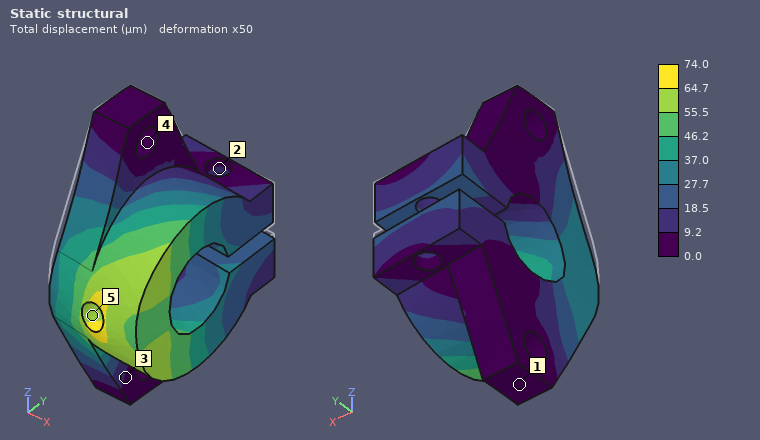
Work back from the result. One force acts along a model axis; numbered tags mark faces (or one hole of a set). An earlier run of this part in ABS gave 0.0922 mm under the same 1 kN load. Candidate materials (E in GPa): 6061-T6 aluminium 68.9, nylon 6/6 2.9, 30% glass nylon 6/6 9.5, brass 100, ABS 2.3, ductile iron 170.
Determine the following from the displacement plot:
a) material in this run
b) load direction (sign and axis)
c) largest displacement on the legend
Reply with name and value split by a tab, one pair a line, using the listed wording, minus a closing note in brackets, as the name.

material in this run	nylon 6/6
load direction	-Z
largest displacement on the legend	74.0 µm
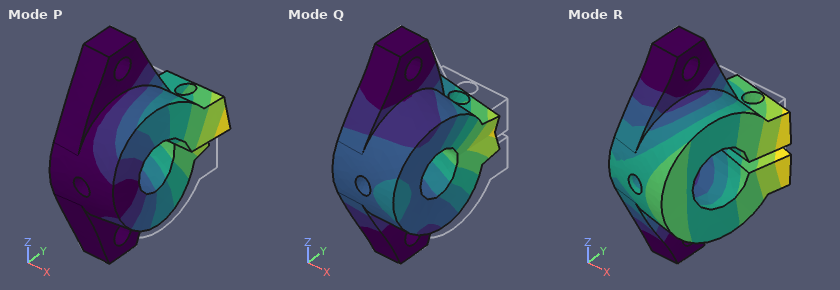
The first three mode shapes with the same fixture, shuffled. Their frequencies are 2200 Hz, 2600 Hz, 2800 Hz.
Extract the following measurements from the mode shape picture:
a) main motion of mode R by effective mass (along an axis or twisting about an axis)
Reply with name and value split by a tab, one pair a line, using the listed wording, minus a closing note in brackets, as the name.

main motion of mode R by effective mass	along Y
